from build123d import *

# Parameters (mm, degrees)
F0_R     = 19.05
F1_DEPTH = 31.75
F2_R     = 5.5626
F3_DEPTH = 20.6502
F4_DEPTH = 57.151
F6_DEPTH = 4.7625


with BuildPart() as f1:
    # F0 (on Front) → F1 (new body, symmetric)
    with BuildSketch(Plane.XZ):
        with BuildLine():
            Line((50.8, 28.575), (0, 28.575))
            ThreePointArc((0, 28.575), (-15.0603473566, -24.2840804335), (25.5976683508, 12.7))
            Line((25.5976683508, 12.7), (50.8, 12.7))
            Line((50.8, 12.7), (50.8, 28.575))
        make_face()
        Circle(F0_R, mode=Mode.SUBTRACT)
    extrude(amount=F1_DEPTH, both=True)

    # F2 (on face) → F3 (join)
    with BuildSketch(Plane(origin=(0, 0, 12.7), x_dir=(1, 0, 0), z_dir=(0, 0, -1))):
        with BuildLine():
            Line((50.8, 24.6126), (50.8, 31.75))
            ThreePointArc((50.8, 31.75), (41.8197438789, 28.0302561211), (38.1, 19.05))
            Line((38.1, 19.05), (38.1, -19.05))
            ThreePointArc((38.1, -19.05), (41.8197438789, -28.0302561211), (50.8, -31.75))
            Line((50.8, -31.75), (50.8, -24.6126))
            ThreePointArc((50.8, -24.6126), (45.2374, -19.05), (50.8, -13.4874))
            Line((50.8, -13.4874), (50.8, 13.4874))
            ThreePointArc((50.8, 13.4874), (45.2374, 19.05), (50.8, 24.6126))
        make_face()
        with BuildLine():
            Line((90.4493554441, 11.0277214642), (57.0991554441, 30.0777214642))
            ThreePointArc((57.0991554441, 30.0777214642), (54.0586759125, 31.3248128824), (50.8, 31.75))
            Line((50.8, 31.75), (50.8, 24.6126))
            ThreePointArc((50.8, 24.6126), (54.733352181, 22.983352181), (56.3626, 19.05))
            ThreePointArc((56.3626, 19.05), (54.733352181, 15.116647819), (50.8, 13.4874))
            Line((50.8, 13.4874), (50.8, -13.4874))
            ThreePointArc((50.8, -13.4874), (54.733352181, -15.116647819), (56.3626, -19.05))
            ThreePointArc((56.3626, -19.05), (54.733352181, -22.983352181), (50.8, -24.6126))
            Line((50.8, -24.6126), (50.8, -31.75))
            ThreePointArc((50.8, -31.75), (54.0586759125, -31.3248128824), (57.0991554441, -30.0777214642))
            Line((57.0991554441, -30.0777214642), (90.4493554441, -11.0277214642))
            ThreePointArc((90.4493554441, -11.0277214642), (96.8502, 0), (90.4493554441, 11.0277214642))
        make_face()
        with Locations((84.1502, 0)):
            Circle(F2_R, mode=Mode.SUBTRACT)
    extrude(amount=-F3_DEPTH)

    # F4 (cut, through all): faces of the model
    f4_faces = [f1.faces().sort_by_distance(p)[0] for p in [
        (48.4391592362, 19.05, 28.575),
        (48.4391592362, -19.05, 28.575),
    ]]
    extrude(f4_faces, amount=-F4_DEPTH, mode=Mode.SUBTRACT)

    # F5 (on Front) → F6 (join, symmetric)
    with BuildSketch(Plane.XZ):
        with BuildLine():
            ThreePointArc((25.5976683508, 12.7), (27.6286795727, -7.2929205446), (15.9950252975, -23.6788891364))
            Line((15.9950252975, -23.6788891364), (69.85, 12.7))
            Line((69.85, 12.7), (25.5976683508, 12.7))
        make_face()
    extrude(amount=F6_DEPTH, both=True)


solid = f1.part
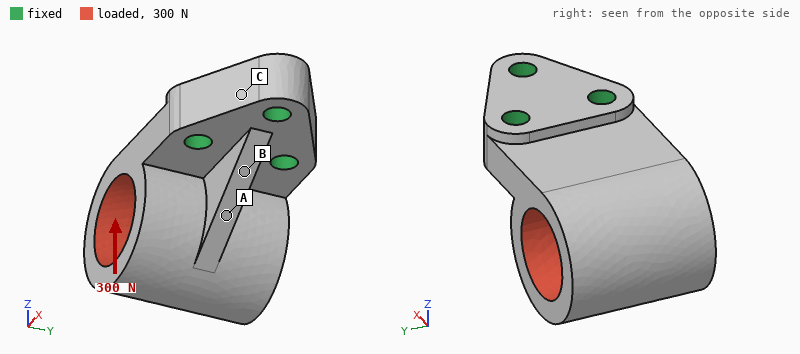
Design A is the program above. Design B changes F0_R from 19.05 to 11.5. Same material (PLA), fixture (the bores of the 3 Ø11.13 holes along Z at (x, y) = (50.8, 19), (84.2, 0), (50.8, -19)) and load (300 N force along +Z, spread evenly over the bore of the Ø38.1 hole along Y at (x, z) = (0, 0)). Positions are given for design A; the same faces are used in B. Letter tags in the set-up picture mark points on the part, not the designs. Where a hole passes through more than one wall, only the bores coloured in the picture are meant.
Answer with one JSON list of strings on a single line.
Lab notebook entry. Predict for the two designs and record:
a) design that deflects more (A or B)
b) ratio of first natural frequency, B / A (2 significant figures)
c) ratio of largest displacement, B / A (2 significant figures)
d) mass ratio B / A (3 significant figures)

["A", "0.91", "0.82", "1.28"]
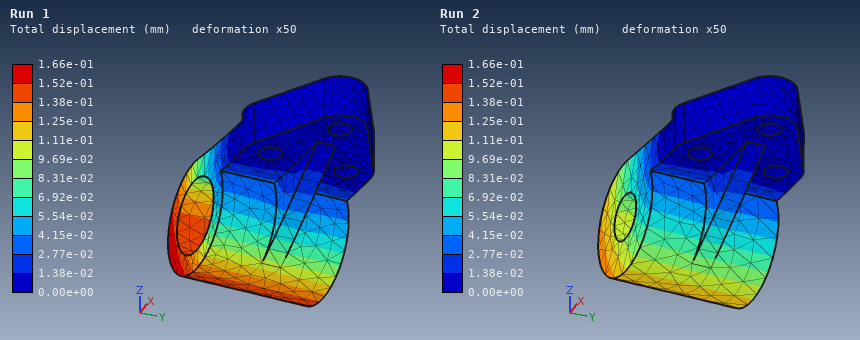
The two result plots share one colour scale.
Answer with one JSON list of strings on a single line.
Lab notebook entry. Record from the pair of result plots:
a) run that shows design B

["Run 2"]
